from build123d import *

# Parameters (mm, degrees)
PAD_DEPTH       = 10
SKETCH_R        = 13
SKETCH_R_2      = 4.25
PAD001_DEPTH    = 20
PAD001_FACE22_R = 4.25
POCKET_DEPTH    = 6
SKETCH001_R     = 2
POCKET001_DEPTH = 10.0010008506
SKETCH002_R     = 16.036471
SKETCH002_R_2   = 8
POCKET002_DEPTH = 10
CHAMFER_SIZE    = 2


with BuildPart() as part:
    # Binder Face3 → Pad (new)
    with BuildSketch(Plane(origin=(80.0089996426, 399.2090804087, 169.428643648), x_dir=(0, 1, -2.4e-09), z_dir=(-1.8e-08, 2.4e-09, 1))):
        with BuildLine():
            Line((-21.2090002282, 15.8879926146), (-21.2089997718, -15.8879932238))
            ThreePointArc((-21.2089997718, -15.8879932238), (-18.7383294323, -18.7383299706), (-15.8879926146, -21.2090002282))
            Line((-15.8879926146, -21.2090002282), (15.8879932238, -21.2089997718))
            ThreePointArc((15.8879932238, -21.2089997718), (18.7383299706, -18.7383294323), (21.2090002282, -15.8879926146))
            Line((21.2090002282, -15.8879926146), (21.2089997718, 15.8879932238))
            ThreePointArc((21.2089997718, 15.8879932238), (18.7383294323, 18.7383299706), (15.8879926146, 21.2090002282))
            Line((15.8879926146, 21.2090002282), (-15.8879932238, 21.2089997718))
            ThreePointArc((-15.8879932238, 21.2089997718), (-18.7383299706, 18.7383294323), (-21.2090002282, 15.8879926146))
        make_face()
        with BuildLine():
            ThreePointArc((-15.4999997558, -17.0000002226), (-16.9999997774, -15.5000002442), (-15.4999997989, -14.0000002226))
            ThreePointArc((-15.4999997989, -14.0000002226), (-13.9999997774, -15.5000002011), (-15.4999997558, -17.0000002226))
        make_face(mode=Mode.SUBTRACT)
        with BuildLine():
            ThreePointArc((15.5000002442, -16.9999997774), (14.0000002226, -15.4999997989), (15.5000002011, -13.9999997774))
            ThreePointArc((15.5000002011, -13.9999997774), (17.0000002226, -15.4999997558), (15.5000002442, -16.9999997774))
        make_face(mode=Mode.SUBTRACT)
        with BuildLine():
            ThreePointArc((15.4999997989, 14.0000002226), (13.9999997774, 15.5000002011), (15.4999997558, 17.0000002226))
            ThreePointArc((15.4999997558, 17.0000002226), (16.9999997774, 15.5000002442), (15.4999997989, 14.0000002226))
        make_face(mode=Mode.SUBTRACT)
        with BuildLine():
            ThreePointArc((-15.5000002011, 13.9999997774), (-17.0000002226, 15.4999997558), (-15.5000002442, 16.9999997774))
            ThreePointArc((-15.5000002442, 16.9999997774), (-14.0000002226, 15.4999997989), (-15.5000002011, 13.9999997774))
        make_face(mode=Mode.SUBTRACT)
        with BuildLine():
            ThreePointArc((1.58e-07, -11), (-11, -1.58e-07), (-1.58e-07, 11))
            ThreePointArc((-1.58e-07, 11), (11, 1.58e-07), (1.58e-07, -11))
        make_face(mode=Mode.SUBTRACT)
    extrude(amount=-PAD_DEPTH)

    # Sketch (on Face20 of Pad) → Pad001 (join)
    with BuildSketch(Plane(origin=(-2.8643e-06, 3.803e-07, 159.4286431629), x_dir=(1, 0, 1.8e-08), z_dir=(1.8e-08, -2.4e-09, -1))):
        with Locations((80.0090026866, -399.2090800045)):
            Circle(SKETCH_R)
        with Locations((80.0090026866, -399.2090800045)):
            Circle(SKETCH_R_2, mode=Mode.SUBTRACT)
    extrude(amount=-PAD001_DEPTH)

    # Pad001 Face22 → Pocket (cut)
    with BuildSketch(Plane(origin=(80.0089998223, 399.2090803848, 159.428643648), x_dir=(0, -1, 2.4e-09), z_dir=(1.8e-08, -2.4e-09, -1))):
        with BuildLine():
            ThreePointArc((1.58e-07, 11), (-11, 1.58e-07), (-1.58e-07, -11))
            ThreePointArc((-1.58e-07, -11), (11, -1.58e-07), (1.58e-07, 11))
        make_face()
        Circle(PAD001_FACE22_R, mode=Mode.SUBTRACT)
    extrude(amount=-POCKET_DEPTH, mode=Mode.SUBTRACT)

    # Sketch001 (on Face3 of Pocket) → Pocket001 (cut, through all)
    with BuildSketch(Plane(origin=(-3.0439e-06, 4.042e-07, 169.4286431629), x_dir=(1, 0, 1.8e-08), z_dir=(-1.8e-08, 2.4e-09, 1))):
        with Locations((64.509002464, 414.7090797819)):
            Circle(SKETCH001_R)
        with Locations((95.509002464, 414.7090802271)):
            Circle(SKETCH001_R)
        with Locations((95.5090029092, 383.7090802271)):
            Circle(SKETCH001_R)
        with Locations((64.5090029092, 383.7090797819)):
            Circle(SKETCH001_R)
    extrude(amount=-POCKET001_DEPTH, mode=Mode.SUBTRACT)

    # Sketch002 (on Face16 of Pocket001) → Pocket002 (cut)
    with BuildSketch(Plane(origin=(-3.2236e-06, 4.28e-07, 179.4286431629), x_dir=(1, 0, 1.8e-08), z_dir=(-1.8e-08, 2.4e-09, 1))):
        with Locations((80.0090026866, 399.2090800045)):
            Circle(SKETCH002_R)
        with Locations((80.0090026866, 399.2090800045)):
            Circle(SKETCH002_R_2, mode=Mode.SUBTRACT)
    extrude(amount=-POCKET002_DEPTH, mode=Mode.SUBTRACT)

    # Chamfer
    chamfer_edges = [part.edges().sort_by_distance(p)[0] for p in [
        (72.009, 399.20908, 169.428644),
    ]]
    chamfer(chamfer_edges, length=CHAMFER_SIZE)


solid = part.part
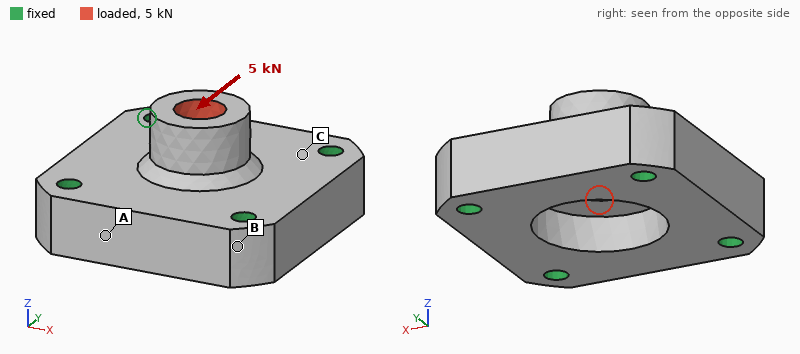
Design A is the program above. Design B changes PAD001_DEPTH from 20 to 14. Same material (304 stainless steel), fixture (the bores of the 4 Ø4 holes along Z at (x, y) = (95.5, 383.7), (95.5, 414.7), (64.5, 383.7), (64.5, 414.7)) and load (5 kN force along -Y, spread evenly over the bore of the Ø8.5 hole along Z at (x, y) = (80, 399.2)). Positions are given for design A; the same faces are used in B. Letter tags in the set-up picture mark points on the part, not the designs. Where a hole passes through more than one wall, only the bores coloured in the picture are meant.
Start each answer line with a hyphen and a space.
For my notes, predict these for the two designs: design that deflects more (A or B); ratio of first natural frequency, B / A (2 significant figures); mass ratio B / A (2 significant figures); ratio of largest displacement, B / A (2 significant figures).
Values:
- A
- 1.1
- 0.95
- 0.47
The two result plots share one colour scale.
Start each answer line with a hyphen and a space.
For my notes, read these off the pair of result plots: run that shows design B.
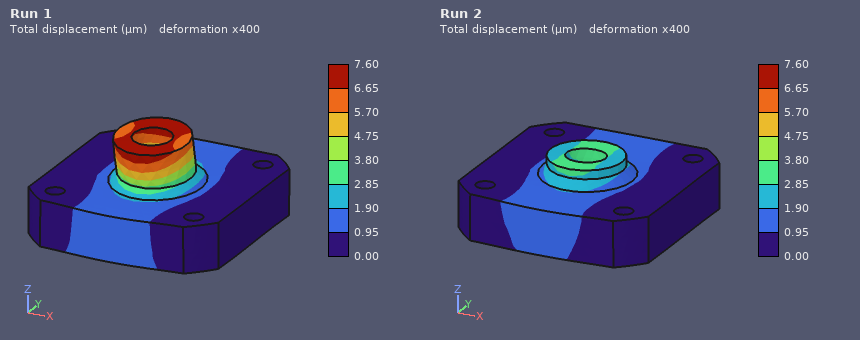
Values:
- Run 2
